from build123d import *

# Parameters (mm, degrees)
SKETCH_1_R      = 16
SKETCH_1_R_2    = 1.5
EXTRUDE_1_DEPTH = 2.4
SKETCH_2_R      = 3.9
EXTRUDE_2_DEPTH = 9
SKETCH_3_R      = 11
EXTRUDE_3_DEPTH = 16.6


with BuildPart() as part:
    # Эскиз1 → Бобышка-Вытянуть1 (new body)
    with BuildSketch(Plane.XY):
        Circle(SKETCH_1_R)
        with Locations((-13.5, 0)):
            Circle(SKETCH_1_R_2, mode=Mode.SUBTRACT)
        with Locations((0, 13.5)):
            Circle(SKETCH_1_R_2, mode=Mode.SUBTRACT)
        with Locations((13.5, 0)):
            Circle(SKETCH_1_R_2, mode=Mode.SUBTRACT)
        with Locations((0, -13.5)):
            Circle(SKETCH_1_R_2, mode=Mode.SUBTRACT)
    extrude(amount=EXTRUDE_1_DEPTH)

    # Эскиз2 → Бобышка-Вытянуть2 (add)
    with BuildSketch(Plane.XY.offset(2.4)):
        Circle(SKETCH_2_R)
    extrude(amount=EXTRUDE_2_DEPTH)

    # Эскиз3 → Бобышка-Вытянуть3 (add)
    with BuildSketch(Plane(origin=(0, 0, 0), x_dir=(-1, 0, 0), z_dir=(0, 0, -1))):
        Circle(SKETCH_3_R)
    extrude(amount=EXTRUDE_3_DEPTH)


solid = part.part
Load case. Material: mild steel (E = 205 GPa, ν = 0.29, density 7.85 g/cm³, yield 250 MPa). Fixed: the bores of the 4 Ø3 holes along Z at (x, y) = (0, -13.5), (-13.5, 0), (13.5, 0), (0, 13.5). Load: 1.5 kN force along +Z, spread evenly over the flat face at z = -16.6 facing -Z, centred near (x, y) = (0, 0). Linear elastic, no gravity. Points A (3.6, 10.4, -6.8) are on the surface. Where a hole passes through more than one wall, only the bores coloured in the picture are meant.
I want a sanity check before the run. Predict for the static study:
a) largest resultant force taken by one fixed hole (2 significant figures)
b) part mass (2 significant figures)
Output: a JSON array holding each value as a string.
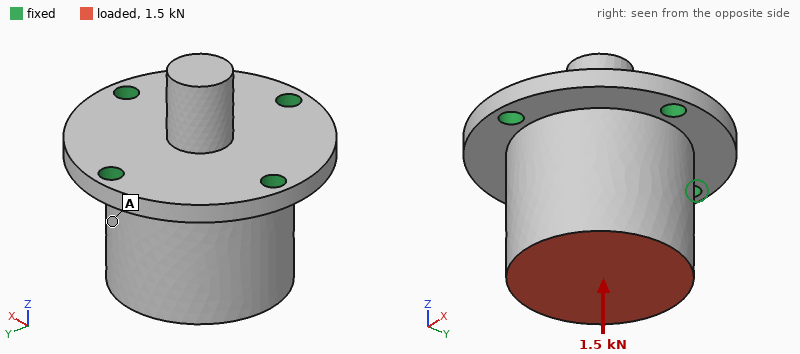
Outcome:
["400 N", "68 g"]
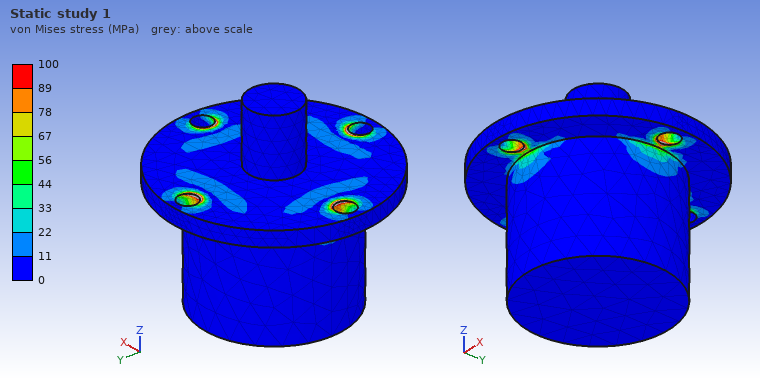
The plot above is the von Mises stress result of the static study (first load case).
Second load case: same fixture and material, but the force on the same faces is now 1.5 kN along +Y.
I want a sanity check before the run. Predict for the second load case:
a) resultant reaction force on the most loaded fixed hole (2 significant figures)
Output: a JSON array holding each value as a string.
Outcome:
["1.2 kN"]
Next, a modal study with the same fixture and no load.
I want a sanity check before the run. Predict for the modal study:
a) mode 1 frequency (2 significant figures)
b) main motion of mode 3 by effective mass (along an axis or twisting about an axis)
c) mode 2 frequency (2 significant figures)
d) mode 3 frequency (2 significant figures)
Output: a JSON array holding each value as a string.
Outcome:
["15 kHz", "along Z", "15 kHz", "20 kHz"]
